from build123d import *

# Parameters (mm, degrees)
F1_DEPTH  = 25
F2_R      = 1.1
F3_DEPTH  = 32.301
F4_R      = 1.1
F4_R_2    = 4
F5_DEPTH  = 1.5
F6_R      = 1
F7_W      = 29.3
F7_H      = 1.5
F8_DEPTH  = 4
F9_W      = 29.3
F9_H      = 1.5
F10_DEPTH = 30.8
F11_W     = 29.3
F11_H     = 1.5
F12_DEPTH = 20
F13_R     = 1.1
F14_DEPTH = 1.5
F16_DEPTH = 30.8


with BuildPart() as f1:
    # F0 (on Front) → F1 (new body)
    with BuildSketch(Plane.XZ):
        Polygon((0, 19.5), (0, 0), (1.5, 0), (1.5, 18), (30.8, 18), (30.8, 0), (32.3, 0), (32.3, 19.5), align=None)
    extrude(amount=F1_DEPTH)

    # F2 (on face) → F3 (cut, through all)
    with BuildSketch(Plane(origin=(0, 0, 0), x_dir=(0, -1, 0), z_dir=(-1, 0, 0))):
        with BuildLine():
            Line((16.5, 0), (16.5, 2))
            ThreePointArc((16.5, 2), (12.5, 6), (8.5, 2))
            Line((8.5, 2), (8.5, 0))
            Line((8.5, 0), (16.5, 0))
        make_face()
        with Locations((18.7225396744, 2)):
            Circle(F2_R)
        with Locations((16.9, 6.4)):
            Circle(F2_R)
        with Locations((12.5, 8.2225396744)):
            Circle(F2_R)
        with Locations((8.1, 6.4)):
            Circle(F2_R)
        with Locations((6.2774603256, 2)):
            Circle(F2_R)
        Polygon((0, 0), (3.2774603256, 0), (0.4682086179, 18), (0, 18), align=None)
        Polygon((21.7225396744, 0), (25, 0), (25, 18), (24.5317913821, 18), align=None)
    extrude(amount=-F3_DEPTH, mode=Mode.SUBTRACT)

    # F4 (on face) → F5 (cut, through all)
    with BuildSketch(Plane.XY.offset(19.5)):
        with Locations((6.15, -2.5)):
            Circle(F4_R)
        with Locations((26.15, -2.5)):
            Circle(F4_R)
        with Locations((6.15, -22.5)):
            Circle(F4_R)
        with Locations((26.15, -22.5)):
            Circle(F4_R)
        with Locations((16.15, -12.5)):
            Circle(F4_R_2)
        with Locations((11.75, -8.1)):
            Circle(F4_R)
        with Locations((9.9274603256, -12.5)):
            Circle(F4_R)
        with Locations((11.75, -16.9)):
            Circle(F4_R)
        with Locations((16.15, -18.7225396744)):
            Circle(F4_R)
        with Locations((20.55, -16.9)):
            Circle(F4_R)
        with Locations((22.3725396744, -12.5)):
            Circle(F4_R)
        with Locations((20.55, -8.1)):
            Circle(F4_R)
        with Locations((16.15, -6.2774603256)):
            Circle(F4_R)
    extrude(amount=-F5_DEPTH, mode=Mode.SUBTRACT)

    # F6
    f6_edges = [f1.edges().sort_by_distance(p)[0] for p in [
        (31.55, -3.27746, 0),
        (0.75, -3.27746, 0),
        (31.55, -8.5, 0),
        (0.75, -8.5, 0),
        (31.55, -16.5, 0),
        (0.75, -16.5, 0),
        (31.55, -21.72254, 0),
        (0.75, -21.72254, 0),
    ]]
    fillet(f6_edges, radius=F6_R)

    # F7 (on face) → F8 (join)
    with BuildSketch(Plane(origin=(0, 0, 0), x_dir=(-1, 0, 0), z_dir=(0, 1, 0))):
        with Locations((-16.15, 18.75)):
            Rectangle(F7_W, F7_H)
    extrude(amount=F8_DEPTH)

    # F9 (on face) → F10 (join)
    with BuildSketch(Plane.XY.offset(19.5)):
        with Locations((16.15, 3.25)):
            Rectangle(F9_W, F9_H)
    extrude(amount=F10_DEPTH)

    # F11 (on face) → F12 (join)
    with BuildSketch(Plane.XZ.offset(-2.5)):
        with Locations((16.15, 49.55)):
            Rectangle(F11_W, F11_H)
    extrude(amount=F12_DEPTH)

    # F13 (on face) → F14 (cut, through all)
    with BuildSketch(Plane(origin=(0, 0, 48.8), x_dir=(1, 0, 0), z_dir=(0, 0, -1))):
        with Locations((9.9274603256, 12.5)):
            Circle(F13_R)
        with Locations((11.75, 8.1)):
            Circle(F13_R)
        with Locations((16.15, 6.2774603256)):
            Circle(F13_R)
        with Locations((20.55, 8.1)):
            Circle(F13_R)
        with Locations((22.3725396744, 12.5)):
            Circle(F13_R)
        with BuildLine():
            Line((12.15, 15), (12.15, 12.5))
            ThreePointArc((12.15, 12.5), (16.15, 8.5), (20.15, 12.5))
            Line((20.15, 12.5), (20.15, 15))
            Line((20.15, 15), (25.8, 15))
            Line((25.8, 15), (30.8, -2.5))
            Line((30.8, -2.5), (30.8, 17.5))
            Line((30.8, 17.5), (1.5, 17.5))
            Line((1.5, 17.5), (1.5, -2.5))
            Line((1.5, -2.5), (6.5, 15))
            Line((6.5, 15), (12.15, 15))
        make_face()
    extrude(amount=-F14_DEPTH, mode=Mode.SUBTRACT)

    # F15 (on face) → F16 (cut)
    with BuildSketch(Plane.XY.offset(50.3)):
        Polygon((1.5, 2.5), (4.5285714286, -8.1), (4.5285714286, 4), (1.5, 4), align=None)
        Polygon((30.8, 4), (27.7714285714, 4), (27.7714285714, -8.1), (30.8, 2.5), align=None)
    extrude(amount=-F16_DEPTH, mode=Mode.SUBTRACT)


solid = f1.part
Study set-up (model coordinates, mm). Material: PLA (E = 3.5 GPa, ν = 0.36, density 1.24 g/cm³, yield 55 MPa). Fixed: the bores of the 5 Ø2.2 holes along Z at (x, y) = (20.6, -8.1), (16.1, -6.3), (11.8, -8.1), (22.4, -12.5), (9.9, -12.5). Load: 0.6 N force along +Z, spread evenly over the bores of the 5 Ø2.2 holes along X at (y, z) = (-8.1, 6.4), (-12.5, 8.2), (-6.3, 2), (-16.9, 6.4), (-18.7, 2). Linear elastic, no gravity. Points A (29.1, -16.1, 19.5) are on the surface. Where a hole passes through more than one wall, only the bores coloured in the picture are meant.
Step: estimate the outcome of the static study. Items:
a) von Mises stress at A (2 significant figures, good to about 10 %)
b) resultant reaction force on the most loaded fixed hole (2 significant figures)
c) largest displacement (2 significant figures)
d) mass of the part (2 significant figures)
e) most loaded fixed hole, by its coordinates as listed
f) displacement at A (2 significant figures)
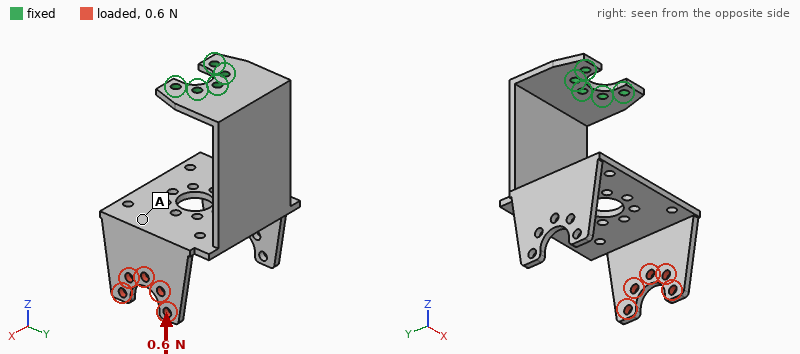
0.19 MPa
0.98 N
0.75 mm
4.7 g
(20.6, -8.1)
0.42 mm
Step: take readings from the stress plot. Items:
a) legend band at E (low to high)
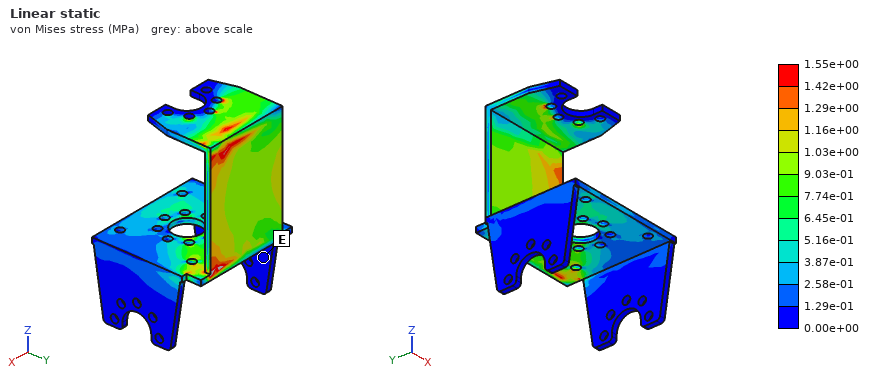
0.00e+00 to 1.29e-01 MPa
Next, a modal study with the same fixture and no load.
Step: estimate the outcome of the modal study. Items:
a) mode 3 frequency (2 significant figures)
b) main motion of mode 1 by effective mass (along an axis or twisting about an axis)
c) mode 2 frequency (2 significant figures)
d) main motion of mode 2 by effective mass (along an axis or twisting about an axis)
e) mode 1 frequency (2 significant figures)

280 Hz
along Y
130 Hz
along X
80 Hz
